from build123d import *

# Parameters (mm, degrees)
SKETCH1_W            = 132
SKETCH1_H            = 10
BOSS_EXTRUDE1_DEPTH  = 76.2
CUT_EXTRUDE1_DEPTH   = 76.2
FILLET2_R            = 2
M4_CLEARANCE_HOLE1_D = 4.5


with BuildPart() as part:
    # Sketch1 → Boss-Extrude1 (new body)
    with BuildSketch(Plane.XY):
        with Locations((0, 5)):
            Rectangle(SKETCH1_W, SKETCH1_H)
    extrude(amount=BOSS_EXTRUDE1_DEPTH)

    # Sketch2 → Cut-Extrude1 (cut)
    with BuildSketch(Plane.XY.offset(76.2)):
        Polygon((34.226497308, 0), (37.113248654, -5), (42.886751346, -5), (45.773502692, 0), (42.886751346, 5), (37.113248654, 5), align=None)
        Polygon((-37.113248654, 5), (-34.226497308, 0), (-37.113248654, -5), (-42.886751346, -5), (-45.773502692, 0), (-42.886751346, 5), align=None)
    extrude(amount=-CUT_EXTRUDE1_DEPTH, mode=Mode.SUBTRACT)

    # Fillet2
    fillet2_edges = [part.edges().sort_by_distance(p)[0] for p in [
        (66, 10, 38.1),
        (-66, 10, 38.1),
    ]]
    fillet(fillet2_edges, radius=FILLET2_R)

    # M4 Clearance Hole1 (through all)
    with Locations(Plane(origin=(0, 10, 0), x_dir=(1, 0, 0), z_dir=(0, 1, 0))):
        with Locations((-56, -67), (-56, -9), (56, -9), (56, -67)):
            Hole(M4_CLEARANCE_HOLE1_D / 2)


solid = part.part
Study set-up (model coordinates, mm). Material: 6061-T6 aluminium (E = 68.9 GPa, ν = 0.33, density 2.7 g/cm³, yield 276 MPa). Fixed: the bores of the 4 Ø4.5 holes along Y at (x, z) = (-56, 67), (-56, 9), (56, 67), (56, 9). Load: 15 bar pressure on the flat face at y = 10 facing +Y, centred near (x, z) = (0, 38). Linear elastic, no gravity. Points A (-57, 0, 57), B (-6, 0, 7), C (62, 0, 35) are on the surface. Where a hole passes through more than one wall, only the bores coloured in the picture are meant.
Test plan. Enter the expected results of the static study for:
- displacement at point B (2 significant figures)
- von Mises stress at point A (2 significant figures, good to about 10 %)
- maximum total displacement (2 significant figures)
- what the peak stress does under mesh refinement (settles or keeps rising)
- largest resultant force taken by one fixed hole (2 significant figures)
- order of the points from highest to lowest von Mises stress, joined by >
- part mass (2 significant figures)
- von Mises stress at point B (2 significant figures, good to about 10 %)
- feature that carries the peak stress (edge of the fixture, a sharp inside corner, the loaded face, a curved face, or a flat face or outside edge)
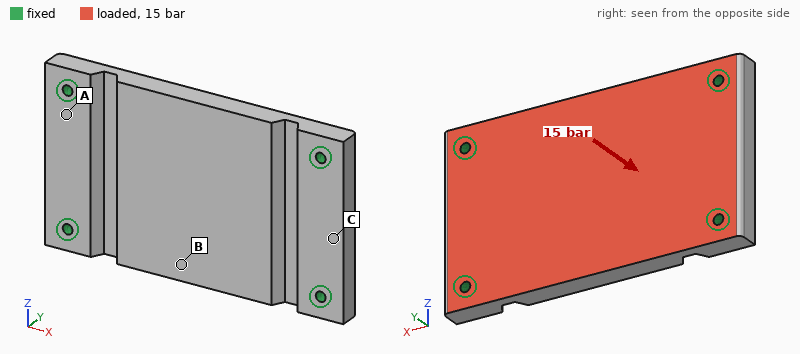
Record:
0.18 mm
38 MPa
0.19 mm
keeps rising
3.7 kN
B > A > C
250 g
67 MPa
edge of the fixture
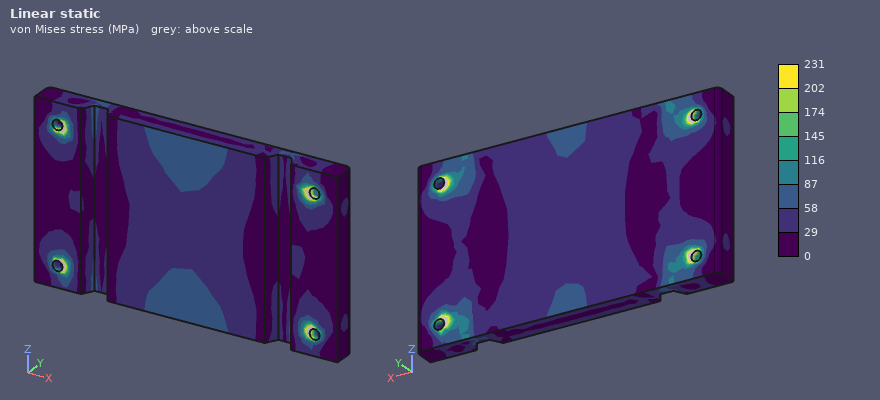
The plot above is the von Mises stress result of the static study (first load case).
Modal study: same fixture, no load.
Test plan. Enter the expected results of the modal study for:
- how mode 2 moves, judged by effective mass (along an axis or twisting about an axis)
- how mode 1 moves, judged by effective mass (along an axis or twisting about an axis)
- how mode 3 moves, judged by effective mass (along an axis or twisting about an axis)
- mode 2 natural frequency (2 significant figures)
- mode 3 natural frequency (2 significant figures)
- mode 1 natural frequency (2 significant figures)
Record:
twisting about X
along Y
twisting about Z
4500 Hz
8000 Hz
3200 Hz
